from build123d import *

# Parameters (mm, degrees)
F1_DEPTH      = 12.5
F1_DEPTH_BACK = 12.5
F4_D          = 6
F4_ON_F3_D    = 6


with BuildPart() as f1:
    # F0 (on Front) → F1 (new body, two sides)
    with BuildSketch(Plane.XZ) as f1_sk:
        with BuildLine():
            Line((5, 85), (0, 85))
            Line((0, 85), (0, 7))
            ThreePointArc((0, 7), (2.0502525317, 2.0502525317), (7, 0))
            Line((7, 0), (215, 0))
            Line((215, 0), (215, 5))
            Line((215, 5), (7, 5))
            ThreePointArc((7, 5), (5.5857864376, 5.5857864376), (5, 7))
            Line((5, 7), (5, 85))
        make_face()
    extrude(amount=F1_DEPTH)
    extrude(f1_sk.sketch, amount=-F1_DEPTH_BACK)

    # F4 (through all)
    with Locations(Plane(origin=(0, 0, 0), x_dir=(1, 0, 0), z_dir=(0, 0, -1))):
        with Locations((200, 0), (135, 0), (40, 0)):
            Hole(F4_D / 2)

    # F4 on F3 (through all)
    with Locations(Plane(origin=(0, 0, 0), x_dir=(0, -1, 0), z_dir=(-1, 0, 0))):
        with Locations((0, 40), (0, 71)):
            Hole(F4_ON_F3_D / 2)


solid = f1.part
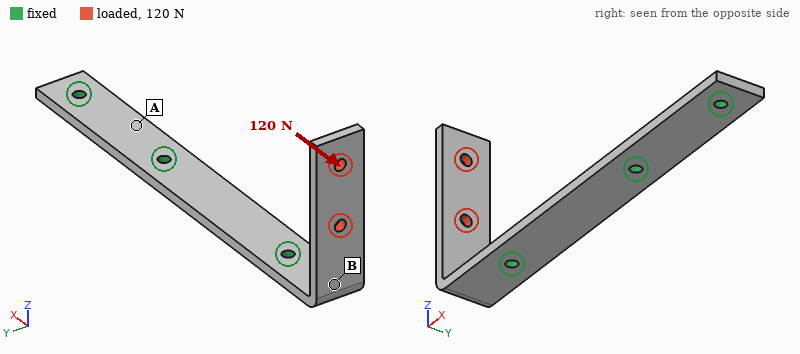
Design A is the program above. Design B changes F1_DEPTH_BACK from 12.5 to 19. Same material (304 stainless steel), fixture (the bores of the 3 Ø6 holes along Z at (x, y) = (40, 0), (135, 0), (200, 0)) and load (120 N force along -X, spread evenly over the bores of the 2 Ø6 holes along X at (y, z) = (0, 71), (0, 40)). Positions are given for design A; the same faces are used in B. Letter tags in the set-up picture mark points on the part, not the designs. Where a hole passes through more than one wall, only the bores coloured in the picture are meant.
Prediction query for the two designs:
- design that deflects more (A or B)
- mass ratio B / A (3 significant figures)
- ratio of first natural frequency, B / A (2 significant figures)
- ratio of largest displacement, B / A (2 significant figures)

A
1.27
0.99
0.81
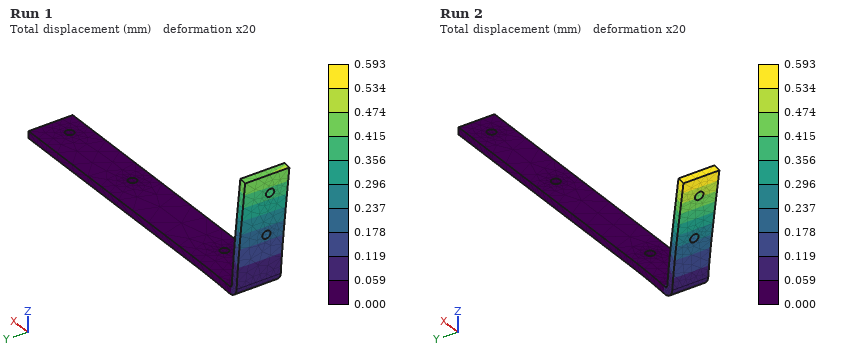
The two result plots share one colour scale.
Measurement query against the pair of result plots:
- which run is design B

Run 1
